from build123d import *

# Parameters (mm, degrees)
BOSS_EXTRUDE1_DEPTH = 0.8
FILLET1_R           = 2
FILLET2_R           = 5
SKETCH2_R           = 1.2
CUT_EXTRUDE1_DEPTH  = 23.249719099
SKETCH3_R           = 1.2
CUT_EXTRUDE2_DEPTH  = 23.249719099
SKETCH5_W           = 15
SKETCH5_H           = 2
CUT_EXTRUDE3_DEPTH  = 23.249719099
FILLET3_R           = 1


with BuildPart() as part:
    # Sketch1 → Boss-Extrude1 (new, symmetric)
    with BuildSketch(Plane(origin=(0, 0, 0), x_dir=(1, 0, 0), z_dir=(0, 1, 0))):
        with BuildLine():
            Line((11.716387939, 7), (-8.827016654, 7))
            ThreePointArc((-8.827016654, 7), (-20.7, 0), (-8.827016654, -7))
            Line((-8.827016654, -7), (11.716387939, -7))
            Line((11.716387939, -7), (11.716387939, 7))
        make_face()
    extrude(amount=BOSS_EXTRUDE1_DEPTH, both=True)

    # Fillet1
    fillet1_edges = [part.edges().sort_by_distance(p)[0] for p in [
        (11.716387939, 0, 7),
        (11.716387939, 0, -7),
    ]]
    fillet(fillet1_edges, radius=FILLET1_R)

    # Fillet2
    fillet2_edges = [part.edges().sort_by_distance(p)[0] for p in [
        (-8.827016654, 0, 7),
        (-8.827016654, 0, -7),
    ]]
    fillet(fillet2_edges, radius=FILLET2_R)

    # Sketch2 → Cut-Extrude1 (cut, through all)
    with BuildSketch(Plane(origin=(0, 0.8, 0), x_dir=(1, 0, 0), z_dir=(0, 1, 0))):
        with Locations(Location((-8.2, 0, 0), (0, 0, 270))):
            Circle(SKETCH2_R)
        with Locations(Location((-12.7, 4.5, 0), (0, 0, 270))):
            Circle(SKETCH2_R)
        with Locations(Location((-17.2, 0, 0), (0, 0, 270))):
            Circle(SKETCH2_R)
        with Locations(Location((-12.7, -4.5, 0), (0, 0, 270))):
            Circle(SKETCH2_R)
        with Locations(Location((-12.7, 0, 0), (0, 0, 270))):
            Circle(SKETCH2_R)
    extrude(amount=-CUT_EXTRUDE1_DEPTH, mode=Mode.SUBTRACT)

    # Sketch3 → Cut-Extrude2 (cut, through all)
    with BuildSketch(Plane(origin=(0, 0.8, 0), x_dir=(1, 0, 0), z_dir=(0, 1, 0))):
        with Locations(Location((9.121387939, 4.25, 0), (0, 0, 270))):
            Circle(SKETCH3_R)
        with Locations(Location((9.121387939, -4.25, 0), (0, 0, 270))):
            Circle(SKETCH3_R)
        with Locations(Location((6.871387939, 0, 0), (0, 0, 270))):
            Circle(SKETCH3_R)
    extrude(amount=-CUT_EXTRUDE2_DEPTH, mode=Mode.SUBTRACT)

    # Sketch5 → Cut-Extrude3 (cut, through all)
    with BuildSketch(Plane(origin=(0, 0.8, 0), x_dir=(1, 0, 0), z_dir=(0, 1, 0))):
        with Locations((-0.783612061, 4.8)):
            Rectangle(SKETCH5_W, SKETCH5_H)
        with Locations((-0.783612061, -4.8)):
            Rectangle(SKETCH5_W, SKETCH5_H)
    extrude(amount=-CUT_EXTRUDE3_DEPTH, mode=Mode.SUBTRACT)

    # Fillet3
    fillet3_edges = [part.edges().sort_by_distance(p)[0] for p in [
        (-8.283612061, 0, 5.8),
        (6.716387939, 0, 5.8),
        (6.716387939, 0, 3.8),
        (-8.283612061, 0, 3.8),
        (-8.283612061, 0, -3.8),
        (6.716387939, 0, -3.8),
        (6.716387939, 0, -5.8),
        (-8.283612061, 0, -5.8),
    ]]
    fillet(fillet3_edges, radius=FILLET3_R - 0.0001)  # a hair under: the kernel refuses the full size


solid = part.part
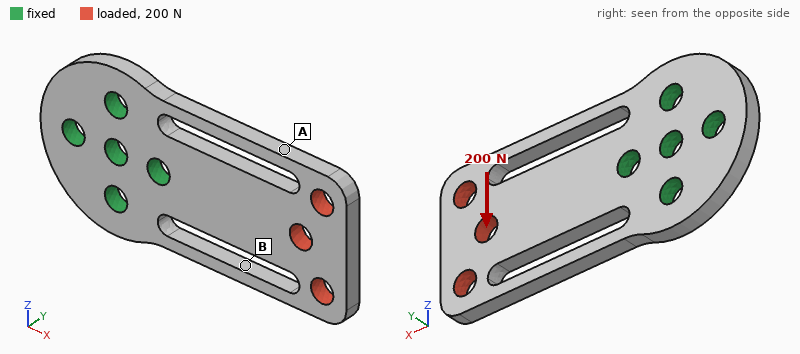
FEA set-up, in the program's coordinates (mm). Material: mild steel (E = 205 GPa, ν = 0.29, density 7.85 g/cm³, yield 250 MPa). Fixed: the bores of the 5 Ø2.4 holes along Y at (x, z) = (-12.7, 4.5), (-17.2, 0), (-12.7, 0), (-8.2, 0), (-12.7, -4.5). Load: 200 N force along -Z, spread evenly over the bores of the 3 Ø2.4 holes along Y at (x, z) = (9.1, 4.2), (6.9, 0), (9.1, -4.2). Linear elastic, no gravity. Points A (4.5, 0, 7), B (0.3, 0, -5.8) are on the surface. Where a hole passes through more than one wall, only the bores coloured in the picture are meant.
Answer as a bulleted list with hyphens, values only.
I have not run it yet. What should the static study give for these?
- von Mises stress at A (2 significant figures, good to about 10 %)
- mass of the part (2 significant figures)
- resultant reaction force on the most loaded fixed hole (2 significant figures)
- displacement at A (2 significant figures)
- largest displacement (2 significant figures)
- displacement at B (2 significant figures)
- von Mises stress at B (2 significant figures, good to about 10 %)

- 19 MPa
- 4.4 g
- 240 N
- 16 µm
- 21 µm
- 11 µm
- 55 MPa
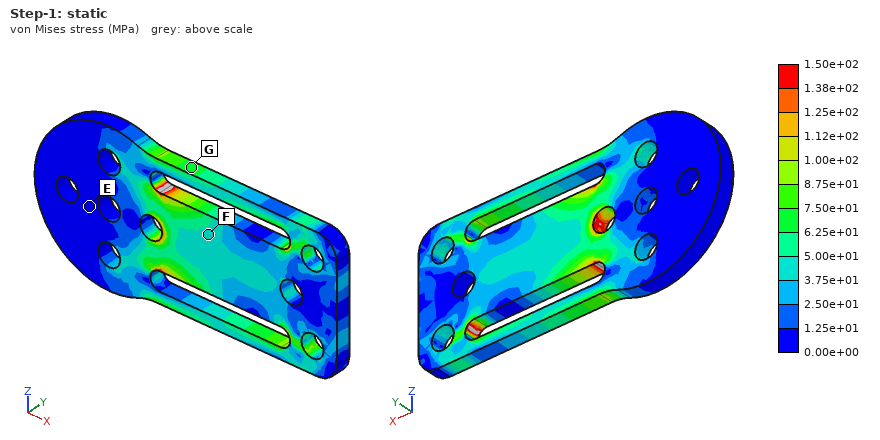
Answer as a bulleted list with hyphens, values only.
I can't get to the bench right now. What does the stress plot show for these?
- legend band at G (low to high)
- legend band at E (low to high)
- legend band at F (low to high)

- 6.25e+01 to 7.50e+01 MPa
- 0.00e+00 to 1.25e+01 MPa
- 3.75e+01 to 5.00e+01 MPa
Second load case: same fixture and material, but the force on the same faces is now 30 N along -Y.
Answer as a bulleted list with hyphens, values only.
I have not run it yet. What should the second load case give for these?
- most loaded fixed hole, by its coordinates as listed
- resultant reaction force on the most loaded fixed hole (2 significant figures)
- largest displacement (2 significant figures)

- (-8.2, 0)
- 63 N
- 80 µm
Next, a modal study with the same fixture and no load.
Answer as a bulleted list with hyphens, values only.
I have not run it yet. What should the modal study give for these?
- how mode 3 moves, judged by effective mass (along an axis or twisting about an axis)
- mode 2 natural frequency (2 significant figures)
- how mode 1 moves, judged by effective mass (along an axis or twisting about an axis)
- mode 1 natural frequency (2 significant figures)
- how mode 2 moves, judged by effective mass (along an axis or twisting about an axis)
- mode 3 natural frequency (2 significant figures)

- along Z
- 8800 Hz
- along Y
- 3300 Hz
- twisting about X
- 14 kHz
